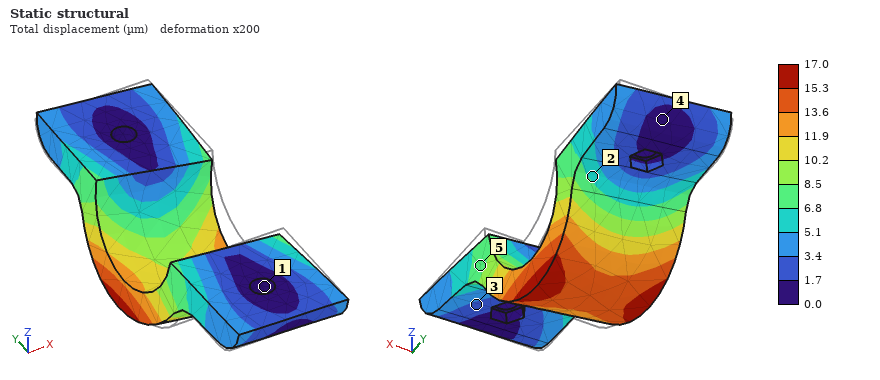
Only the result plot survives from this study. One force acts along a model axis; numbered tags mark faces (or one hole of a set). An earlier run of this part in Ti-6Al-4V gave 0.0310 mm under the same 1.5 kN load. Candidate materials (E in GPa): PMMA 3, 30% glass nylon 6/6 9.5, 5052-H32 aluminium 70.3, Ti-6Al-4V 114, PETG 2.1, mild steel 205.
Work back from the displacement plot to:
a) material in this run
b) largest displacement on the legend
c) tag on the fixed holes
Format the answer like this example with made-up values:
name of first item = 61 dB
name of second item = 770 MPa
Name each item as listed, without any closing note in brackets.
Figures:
material in this run = mild steel
largest displacement on the legend = 17.0 µm
tag on the fixed holes = 1
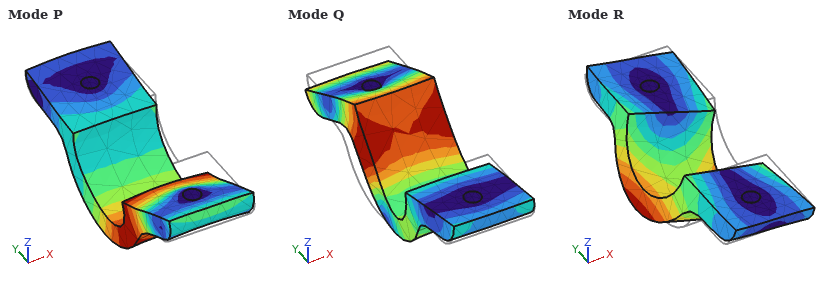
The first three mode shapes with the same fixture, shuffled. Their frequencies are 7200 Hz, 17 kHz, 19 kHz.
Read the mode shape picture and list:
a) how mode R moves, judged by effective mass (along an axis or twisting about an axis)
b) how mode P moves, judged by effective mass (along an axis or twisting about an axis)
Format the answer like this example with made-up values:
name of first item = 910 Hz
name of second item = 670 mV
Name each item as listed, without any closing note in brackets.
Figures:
how mode R moves, judged by effective mass = along X
how mode P moves, judged by effective mass = along Z
